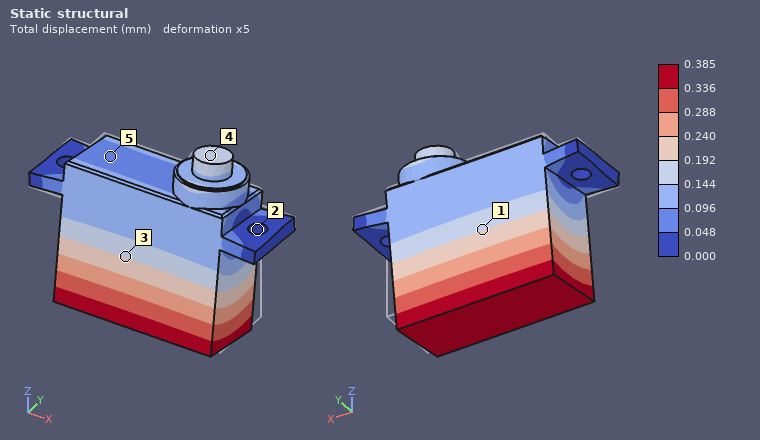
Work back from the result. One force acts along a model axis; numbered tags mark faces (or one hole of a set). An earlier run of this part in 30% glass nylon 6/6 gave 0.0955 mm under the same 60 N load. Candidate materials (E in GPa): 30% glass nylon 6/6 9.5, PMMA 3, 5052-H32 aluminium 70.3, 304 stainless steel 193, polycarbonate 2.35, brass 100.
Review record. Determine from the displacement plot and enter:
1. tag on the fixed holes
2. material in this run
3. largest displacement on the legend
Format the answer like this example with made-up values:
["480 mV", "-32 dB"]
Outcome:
["2", "polycarbonate", "0.385 mm"]
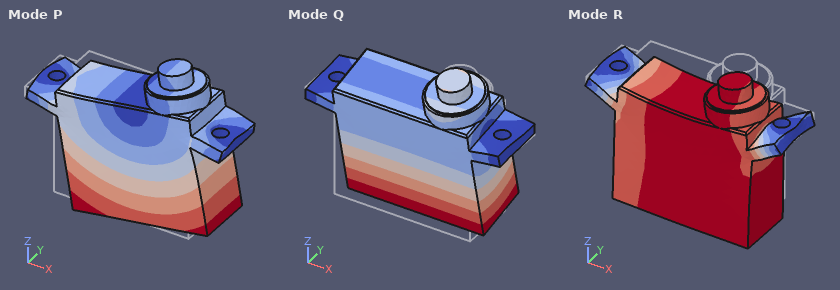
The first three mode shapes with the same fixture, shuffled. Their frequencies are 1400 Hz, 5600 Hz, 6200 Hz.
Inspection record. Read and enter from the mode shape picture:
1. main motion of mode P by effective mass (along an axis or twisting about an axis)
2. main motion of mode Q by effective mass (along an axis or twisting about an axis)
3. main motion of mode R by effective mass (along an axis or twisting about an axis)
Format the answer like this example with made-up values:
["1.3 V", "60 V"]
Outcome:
["along X", "along Y", "along Z"]
